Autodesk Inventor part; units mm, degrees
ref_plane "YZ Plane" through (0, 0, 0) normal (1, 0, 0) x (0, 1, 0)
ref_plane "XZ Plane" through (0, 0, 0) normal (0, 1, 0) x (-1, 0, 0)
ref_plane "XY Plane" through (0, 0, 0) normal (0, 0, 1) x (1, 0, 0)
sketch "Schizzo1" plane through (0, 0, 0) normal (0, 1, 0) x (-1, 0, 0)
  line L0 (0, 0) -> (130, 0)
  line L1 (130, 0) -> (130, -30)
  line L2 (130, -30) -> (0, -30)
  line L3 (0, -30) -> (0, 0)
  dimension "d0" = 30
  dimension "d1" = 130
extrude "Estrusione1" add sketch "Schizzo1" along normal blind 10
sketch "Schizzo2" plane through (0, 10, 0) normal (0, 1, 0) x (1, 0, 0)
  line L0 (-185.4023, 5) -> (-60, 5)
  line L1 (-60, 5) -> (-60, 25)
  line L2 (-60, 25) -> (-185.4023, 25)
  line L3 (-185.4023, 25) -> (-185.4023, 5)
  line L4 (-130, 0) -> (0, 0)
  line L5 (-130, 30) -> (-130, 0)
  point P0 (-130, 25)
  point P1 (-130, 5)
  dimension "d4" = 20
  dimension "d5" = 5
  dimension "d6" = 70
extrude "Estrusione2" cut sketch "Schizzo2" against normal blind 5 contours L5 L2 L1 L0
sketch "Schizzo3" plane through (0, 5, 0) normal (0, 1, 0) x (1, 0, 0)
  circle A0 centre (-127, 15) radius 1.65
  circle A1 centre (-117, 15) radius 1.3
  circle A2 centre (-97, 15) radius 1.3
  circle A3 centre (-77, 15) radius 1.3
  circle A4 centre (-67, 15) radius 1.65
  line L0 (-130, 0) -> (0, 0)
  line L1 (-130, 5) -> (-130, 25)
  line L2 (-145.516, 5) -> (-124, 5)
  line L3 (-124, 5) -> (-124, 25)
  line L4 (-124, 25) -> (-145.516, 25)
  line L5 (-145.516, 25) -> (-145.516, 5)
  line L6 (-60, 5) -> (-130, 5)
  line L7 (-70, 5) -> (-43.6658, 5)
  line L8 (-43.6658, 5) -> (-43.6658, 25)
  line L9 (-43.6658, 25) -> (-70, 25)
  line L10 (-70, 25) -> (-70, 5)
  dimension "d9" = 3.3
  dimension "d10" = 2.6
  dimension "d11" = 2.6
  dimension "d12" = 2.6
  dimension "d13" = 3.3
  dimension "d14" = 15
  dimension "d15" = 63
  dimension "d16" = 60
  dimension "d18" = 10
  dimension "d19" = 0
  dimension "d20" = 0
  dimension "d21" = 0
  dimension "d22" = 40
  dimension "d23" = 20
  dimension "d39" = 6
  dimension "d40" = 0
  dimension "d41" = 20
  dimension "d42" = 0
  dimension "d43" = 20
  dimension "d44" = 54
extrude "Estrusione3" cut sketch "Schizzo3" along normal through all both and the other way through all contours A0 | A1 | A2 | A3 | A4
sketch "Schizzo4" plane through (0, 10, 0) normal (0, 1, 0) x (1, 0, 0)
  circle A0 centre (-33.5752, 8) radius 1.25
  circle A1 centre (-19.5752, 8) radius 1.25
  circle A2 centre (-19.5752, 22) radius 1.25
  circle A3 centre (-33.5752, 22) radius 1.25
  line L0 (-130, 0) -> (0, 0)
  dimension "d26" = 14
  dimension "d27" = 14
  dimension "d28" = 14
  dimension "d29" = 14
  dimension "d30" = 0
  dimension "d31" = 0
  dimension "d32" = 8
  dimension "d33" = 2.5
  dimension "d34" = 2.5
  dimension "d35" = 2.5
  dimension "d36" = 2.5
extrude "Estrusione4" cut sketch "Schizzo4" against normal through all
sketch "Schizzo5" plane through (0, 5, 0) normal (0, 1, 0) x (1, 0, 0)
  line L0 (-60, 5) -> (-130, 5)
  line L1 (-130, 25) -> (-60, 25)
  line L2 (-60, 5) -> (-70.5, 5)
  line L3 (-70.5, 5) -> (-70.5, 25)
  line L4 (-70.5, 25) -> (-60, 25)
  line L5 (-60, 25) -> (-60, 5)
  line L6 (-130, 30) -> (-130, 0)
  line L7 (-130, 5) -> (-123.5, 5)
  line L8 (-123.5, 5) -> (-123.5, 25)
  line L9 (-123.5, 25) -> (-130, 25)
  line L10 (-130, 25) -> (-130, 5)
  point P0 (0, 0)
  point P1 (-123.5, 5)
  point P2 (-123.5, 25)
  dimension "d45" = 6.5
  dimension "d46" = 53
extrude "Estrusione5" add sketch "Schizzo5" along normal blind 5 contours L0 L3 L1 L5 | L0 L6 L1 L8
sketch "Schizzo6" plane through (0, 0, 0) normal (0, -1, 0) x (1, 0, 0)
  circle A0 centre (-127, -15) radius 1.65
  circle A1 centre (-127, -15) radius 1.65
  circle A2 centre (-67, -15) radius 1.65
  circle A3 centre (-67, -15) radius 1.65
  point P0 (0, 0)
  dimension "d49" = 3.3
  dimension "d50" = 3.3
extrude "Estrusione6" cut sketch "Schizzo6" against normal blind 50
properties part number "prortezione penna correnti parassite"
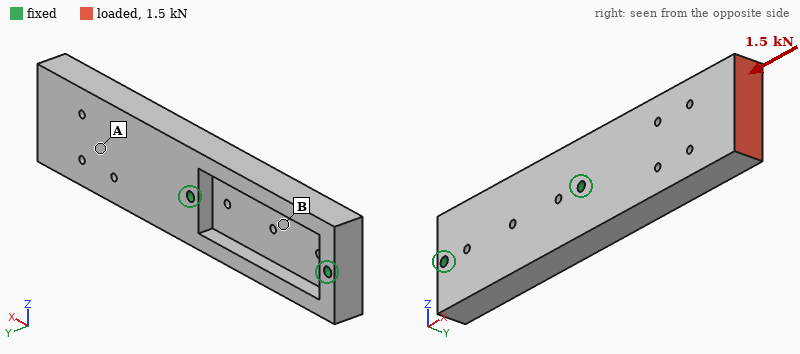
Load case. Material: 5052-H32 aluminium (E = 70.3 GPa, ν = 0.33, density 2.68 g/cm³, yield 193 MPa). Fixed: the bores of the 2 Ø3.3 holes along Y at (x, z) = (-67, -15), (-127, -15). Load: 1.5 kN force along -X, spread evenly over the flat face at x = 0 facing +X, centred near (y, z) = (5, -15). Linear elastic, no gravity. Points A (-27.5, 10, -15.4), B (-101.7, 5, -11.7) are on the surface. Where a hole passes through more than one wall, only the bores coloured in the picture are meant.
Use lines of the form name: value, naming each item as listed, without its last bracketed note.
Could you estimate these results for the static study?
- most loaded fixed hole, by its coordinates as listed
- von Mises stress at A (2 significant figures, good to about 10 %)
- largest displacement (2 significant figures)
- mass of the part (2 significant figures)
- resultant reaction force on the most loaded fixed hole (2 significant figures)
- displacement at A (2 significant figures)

most loaded fixed hole, by its coordinates as listed: (-67, -15)
von Mises stress at A: 5.6 MPa
largest displacement: 5.9 µm
mass of the part: 89 g
resultant reaction force on the most loaded fixed hole: 1.3 kN
displacement at A: 3.8 µm
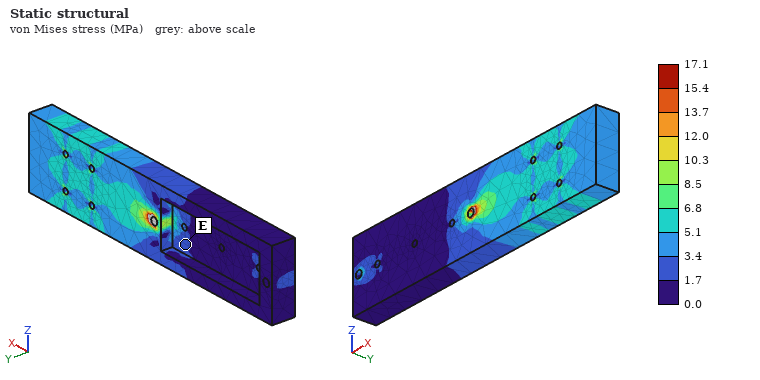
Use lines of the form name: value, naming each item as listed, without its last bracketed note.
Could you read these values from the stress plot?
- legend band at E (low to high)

legend band at E: 1.7 to 3.4 MPa
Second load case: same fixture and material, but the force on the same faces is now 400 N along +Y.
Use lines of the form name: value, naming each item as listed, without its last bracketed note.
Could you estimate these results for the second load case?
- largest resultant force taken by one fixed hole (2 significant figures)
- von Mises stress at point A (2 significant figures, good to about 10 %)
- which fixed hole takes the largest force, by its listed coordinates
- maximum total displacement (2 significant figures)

largest resultant force taken by one fixed hole: 520 N
von Mises stress at point A: 23 MPa
which fixed hole takes the largest force, by its listed coordinates: (-67, -15)
maximum total displacement: 0.28 mm
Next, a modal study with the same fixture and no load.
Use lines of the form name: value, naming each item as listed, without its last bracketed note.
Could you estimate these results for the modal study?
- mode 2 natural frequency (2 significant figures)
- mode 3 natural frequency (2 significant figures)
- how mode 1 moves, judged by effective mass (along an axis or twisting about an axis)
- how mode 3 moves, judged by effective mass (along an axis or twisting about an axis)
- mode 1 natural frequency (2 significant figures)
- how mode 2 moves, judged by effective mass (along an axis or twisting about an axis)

mode 2 natural frequency: 3200 Hz
mode 3 natural frequency: 6000 Hz
how mode 1 moves, judged by effective mass: along Y
how mode 3 moves, judged by effective mass: twisting about X
mode 1 natural frequency: 1600 Hz
how mode 2 moves, judged by effective mass: along Z
